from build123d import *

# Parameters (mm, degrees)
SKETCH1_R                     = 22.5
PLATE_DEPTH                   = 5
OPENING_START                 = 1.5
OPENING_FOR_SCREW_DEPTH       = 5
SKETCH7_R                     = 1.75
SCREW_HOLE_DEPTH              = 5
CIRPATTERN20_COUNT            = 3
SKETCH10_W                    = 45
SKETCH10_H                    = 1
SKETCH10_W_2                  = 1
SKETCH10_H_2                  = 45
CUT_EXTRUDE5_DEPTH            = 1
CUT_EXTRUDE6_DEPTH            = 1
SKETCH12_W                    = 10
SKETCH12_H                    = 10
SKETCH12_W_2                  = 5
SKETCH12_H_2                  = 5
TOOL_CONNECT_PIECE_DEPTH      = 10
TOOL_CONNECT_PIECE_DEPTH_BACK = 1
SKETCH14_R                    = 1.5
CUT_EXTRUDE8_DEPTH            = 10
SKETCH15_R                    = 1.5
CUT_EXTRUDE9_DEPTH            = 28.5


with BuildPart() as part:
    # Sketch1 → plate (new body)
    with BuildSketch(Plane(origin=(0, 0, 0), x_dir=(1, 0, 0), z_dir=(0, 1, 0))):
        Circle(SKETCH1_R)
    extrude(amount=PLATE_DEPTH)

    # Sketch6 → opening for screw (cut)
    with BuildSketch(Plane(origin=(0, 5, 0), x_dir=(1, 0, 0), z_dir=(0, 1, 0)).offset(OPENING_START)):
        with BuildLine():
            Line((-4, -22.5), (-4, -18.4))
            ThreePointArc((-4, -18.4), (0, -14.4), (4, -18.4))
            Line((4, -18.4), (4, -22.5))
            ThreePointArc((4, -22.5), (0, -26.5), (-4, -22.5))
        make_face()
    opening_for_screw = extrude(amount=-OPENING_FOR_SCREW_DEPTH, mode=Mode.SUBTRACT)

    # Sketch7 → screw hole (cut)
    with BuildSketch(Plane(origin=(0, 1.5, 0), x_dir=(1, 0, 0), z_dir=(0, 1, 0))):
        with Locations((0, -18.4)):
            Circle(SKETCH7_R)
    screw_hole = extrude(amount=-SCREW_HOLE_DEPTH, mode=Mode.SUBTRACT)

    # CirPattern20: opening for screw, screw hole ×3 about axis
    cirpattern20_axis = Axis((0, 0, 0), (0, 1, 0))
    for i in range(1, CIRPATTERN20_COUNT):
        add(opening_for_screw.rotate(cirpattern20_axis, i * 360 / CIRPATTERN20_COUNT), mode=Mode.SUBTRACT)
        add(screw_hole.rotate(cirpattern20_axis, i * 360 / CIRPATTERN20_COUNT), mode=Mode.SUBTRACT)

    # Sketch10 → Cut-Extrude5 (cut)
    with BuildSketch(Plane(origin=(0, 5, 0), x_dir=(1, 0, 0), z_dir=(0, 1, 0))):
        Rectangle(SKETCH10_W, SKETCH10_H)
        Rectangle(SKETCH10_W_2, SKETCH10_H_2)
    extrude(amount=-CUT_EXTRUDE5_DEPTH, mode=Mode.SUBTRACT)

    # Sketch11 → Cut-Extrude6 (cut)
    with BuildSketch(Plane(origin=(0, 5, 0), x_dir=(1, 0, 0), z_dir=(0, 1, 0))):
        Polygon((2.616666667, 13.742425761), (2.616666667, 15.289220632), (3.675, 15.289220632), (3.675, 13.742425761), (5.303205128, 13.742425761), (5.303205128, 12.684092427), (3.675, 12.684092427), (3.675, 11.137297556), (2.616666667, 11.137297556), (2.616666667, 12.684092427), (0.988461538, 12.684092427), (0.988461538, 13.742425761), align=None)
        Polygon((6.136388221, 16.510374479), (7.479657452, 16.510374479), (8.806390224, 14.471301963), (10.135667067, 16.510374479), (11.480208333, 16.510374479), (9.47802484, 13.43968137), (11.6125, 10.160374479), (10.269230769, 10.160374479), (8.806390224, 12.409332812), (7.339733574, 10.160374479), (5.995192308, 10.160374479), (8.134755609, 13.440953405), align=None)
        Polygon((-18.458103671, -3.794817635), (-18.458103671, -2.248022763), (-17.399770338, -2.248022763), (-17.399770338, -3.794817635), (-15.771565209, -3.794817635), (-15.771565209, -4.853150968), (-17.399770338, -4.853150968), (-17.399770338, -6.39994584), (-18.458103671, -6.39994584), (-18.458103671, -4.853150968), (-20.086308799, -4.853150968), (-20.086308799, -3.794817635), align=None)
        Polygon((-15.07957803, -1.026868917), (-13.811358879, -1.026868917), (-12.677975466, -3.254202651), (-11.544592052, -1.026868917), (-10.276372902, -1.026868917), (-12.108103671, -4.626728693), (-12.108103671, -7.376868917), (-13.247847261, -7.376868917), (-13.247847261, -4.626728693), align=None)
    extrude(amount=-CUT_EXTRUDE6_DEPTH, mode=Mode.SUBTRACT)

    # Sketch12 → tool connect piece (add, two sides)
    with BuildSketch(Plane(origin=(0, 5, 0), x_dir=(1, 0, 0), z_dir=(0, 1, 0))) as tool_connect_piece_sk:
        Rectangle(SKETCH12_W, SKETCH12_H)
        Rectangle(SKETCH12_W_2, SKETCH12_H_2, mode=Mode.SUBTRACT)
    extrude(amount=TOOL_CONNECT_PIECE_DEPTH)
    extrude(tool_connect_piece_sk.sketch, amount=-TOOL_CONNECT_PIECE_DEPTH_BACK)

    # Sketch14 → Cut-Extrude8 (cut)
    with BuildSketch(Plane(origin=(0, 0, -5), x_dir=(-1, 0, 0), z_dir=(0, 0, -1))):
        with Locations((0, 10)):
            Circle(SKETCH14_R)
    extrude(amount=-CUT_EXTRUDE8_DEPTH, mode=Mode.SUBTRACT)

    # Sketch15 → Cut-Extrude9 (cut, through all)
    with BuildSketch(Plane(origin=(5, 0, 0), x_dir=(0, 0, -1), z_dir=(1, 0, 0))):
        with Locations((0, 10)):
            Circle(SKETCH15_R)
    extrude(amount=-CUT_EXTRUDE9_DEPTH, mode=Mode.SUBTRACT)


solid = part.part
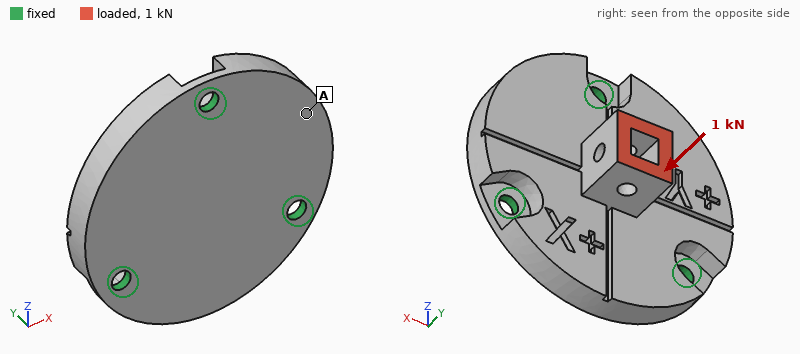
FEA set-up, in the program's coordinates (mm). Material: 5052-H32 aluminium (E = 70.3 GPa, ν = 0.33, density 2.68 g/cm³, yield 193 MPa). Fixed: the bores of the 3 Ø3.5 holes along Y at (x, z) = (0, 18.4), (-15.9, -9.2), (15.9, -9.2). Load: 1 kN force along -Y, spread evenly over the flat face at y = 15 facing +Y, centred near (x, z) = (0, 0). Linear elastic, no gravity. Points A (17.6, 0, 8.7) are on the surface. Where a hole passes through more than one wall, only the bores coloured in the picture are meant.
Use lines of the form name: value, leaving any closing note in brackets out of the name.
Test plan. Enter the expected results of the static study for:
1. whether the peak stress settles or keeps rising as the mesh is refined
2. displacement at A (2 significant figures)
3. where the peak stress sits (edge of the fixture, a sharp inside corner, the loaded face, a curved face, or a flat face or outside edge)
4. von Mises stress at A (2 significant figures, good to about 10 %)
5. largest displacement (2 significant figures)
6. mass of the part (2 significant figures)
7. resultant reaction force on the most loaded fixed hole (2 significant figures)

whether the peak stress settles or keeps rising as the mesh is refined: keeps rising
displacement at A: 7.1 µm
where the peak stress sits: edge of the fixture
von Mises stress at A: 11 MPa
largest displacement: 19 µm
mass of the part: 21 g
resultant reaction force on the most loaded fixed hole: 470 N
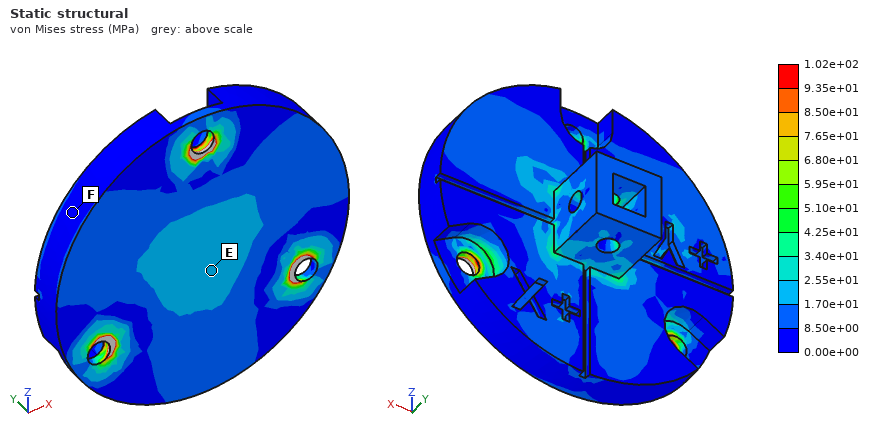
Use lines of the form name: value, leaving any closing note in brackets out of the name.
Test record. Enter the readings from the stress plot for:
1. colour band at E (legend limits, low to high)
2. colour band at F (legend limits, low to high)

colour band at E: 1.70e+01 to 2.55e+01 MPa
colour band at F: 0.00e+00 to 8.50e+00 MPa
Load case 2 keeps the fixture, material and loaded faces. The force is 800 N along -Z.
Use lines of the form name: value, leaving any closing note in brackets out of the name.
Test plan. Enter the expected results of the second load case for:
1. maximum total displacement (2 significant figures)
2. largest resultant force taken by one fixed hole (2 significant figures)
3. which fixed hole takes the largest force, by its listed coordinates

maximum total displacement: 43 µm
largest resultant force taken by one fixed hole: 700 N
which fixed hole takes the largest force, by its listed coordinates: (0, 18.4)
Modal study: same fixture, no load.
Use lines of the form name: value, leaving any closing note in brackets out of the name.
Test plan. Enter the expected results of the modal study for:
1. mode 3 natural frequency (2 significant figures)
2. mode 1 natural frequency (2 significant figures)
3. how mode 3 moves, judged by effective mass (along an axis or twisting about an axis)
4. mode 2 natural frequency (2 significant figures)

mode 3 natural frequency: 11 kHz
mode 1 natural frequency: 10 kHz
how mode 3 moves, judged by effective mass: along Y
mode 2 natural frequency: 10 kHz
